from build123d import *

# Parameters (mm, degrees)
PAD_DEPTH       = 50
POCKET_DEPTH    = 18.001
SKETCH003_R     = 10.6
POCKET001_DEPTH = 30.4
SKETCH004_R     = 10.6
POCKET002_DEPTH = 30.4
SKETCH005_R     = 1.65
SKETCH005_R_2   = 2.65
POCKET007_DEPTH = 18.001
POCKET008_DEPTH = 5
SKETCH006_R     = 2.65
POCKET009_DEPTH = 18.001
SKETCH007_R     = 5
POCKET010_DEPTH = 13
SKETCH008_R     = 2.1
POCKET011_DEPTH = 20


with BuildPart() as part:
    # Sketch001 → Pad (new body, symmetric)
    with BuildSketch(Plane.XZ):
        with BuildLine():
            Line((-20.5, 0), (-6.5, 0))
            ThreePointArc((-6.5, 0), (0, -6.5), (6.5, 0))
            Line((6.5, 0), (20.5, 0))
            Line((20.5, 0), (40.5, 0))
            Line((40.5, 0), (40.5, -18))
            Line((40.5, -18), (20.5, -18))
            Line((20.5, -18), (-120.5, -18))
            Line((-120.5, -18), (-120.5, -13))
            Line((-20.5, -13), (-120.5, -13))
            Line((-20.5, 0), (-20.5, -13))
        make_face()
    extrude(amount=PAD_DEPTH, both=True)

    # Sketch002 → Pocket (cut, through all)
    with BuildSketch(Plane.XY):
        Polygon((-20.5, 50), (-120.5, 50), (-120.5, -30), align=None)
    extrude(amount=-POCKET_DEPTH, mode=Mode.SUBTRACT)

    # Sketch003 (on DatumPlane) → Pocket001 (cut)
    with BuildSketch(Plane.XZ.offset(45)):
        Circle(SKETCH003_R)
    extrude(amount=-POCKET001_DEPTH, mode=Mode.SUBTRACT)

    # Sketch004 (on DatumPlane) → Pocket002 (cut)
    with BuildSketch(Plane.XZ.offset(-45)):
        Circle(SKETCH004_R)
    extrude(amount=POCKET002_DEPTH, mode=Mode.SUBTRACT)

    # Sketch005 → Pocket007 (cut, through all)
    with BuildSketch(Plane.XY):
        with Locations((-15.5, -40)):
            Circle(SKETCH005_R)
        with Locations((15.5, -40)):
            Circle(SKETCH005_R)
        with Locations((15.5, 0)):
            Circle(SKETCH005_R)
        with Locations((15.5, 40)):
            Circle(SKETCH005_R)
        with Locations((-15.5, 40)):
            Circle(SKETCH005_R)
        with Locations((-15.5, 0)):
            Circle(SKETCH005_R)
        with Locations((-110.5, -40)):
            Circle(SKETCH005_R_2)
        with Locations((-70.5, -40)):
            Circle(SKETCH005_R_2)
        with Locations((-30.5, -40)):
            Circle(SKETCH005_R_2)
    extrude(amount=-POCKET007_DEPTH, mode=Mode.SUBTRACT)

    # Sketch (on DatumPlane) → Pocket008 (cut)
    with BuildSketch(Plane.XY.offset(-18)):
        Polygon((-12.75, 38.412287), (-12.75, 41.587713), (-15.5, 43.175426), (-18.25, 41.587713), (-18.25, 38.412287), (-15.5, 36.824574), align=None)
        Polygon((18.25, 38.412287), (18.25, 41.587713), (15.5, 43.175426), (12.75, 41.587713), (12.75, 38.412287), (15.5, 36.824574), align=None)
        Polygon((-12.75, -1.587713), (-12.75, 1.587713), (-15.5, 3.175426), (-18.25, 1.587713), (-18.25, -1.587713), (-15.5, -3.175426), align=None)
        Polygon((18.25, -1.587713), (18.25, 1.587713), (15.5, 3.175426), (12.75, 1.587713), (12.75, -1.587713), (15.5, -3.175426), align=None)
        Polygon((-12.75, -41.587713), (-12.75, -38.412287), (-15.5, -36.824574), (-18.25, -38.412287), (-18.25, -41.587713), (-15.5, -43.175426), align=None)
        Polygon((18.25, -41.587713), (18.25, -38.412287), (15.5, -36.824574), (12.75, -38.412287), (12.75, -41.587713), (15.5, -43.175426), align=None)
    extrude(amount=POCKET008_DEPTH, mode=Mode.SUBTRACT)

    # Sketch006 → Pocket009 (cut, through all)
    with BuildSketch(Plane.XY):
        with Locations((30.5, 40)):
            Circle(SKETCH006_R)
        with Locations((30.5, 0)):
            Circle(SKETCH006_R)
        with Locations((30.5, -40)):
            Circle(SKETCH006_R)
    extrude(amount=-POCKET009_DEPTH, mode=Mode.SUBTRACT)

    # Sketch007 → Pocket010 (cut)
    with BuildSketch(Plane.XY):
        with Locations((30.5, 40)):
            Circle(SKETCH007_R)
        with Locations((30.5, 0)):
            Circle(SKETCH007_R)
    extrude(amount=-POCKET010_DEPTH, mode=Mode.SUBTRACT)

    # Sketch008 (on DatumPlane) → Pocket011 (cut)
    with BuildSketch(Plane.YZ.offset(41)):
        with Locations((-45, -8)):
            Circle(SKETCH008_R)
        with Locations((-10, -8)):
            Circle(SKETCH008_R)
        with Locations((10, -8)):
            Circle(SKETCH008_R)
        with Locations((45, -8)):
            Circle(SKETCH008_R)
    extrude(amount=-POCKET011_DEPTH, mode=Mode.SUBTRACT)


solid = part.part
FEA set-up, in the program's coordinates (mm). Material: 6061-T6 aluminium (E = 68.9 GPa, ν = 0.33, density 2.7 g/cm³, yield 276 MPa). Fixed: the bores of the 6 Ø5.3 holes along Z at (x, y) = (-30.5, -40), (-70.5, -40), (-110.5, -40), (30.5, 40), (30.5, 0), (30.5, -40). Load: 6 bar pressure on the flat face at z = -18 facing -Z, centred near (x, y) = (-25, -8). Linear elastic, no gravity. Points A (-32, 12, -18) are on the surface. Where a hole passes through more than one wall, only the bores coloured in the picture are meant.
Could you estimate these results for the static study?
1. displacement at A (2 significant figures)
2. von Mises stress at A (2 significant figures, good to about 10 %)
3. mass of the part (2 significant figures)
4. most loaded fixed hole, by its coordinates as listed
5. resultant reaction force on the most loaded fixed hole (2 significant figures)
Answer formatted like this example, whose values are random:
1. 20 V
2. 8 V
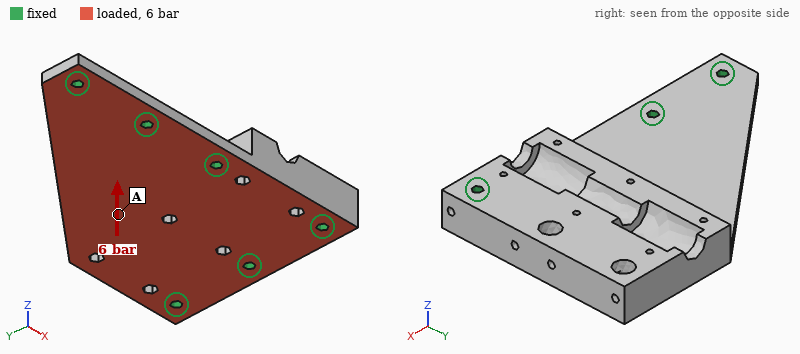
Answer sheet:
1. 0.16 mm
2. 20 MPa
3. 330 g
4. (-30.5, -40)
5. 2.7 kN
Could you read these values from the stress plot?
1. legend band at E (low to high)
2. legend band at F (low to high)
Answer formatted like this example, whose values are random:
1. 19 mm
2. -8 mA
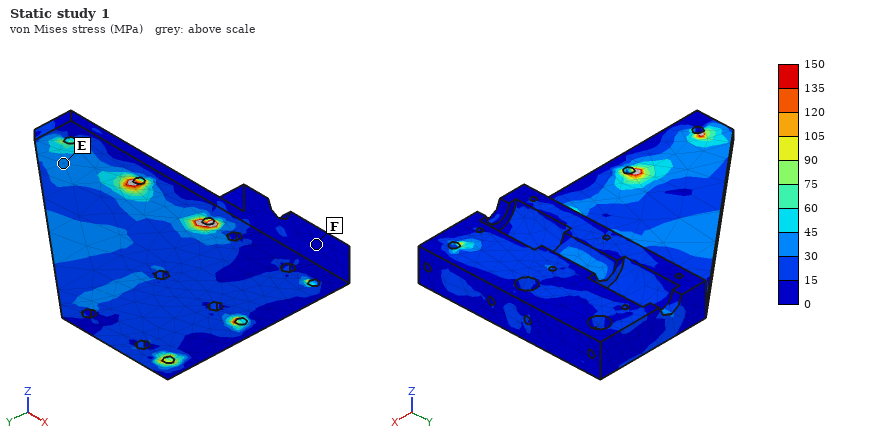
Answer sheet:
1. 30 to 45 MPa
2. 0 to 15 MPa
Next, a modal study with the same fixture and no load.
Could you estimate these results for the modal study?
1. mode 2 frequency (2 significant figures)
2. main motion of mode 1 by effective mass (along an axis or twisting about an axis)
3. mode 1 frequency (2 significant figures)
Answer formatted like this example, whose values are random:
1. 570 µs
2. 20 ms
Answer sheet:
1. 3700 Hz
2. along Z
3. 2300 Hz
